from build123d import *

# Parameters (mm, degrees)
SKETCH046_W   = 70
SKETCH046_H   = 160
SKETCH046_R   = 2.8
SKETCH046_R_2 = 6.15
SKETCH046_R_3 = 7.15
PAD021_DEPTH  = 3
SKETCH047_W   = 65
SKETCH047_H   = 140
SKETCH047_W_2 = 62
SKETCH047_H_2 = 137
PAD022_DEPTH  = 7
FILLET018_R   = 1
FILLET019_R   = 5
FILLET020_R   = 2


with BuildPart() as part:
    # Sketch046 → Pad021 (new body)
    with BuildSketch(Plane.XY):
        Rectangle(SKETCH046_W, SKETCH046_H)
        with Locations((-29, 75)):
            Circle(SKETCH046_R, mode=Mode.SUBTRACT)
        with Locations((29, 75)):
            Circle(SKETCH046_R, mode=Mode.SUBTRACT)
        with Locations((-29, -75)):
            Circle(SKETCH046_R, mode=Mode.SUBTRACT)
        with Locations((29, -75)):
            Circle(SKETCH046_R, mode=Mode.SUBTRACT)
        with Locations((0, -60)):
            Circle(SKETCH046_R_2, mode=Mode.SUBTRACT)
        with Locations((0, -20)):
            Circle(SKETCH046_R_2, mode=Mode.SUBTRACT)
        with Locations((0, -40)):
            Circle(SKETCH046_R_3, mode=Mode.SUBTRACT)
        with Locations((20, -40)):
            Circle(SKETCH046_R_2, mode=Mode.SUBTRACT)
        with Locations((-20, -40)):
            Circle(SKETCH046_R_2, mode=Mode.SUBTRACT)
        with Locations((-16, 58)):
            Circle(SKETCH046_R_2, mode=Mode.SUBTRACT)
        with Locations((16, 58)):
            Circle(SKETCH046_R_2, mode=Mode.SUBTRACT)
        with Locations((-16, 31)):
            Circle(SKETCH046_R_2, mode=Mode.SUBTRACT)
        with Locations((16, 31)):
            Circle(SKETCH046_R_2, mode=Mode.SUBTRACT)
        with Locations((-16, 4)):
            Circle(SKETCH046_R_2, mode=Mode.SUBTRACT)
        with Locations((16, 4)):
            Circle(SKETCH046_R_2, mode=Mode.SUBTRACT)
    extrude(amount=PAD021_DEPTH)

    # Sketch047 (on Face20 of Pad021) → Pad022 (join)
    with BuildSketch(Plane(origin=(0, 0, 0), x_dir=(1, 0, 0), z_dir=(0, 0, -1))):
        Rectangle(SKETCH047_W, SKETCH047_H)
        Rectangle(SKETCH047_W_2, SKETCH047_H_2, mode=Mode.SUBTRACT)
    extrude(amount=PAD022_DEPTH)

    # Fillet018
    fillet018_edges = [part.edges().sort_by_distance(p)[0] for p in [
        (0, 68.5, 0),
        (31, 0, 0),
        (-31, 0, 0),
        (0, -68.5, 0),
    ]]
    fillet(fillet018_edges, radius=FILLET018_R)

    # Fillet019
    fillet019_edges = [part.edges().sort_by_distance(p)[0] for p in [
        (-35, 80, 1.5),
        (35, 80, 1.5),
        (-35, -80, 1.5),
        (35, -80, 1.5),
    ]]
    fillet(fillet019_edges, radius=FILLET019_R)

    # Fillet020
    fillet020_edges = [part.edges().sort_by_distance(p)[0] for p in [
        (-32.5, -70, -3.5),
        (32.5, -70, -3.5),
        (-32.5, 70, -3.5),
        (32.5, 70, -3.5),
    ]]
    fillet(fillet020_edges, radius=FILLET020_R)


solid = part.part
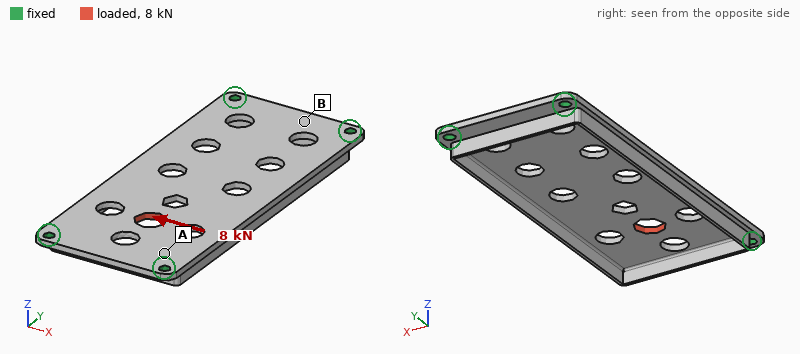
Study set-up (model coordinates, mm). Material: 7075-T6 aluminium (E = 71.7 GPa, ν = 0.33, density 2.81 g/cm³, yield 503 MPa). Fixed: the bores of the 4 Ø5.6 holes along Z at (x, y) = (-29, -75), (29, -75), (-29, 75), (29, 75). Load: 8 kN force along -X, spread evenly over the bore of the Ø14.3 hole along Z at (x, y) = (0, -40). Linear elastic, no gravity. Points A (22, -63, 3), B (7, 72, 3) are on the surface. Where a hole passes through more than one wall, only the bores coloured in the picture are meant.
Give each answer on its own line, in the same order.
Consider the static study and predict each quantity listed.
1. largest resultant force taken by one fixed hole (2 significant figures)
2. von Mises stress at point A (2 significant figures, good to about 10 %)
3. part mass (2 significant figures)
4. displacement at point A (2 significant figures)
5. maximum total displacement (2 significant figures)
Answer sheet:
3.8 kN
76 MPa
94 g
0.025 mm
0.11 mm
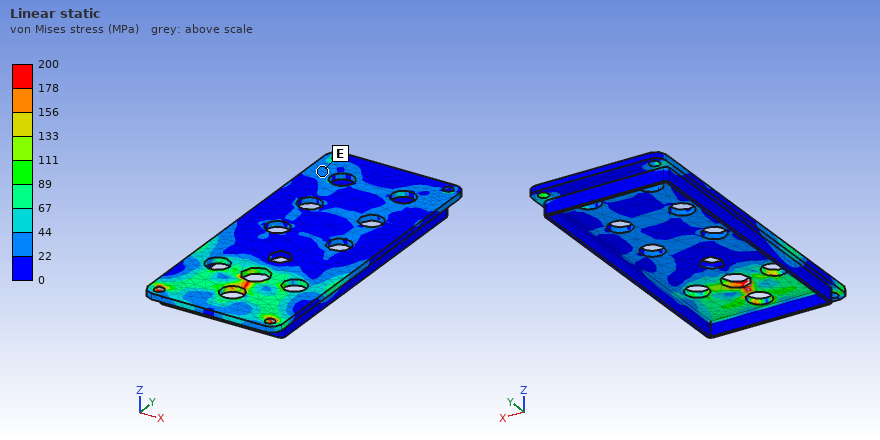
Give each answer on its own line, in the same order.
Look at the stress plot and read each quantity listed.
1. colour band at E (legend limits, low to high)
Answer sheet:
22 to 44 MPa
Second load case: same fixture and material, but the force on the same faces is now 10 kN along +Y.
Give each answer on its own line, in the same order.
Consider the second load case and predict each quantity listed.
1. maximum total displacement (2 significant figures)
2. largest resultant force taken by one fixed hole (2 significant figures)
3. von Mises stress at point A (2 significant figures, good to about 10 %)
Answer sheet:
55 µm
3.9 kN
73 MPa
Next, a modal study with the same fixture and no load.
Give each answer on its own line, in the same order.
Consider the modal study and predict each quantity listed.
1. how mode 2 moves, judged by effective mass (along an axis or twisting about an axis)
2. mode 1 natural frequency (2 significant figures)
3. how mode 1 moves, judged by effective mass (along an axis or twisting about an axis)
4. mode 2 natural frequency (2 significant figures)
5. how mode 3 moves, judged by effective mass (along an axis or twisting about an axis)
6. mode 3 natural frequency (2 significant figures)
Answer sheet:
twisting about Y
980 Hz
along Z
1500 Hz
twisting about X
2600 Hz
